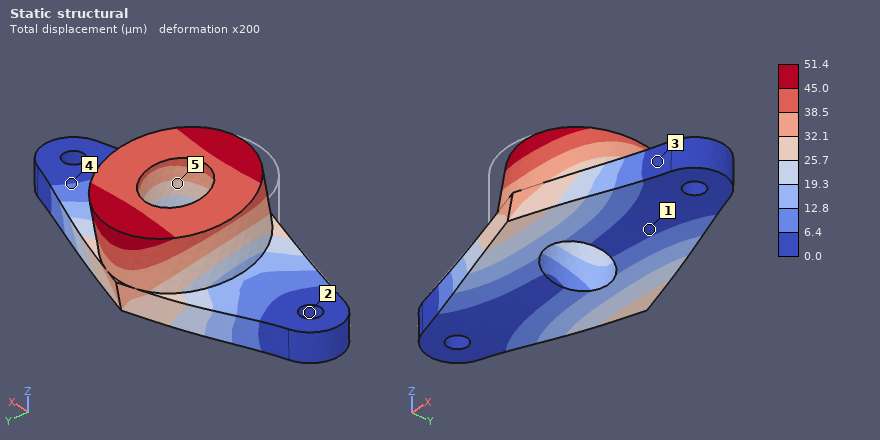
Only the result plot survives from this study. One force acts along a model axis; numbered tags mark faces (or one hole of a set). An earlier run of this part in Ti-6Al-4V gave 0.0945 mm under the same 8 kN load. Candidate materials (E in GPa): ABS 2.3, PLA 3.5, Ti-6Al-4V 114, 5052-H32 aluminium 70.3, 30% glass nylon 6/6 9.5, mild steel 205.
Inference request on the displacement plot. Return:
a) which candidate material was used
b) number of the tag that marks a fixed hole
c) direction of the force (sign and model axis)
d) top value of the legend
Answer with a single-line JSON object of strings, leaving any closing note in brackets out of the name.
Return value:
{"which candidate material was used": "mild steel", "number of the tag that marks a fixed hole": "2", "direction of the force": "+Y", "top value of the legend": "51.4 µm"}
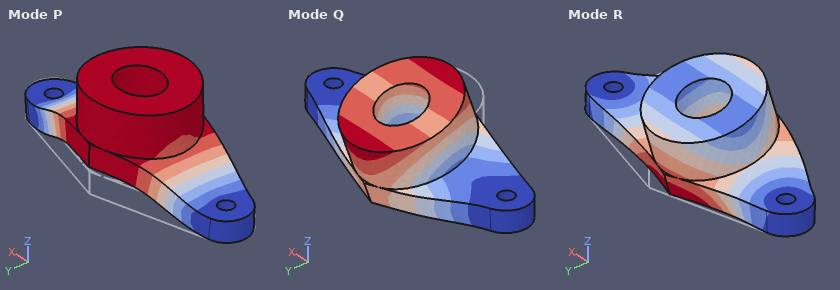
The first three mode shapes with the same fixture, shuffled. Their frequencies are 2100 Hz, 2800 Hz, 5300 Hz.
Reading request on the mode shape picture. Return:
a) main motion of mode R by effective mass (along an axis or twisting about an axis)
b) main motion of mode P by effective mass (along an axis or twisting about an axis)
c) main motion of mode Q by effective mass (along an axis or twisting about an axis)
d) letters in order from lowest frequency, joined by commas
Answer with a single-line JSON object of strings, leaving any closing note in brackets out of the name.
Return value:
{"main motion of mode R by effective mass": "along Y", "main motion of mode P by effective mass": "along Z", "main motion of mode Q by effective mass": "along Y", "letters in order from lowest frequency, joined by commas": "Q, P, R"}
